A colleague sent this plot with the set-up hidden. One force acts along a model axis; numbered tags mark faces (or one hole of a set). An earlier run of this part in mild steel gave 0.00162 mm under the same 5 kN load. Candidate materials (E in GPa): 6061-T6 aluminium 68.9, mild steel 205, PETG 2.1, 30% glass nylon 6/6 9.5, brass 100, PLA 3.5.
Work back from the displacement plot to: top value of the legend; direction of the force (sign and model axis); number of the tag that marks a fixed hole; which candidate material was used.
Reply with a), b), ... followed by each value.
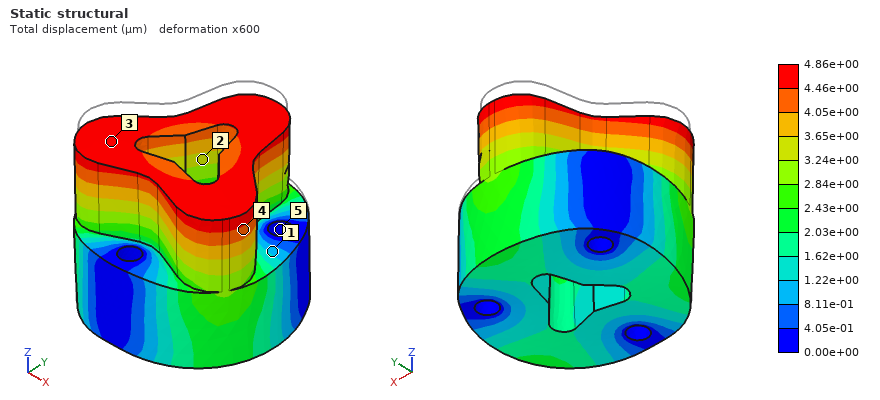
a) 4.86e+00 µm
b) -Z
c) 5
d) 6061-T6 aluminium
